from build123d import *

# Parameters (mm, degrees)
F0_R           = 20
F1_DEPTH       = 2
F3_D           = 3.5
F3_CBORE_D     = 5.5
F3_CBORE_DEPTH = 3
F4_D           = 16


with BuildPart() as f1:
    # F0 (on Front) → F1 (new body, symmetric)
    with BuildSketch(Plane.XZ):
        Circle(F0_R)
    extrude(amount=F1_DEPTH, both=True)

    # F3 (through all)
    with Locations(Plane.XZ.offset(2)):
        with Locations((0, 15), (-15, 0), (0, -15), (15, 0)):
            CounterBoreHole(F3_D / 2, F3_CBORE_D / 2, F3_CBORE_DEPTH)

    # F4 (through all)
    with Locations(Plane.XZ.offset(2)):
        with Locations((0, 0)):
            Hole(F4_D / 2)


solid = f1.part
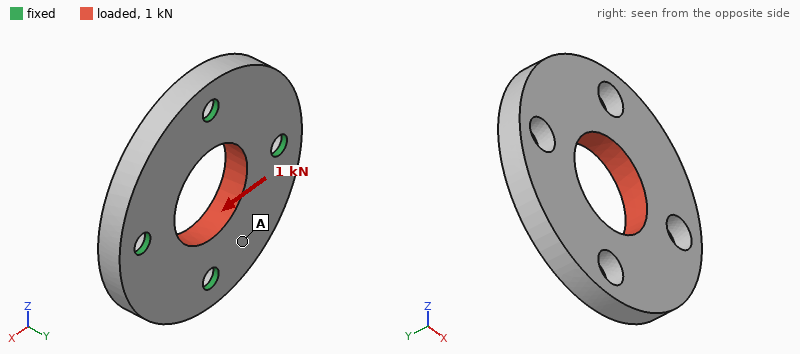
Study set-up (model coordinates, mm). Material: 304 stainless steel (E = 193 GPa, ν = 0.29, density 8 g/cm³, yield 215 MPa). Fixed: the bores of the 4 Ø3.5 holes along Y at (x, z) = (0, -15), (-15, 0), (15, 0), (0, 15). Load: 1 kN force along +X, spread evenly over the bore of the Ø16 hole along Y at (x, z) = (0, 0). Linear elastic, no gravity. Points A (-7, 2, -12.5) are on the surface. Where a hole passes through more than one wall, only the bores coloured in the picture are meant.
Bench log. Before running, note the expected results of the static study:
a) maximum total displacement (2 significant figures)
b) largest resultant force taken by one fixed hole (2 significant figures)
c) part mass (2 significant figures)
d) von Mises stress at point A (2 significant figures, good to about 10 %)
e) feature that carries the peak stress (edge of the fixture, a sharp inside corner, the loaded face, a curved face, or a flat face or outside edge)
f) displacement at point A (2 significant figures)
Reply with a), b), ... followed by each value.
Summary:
a) 1.1 µm
b) 270 N
c) 31 g
d) 6.2 MPa
e) edge of the fixture
f) 0.48 µm
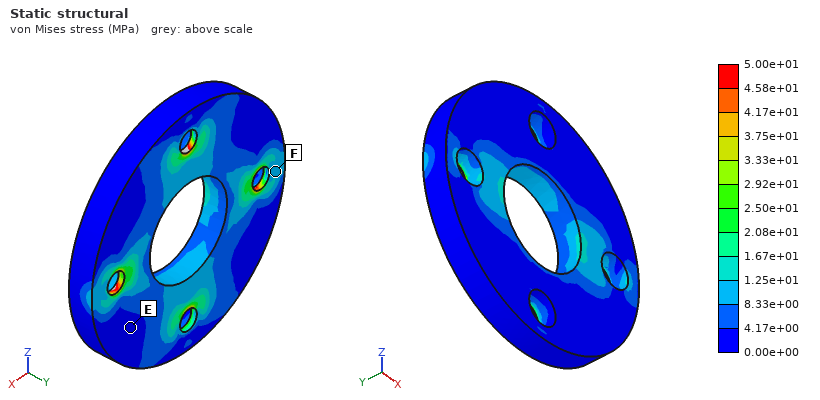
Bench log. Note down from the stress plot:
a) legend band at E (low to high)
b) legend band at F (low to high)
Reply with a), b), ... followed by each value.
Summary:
a) 0.00e+00 to 4.17e+00 MPa
b) 8.33e+00 to 1.25e+01 MPa
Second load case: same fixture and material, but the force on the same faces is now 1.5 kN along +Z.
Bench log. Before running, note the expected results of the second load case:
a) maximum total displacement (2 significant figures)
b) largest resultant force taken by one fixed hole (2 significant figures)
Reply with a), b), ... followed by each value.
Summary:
a) 1.6 µm
b) 400 N
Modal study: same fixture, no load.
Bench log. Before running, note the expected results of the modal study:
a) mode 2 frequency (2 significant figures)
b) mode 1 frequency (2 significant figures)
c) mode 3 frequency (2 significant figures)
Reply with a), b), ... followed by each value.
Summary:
a) 19 kHz
b) 16 kHz
c) 19 kHz
